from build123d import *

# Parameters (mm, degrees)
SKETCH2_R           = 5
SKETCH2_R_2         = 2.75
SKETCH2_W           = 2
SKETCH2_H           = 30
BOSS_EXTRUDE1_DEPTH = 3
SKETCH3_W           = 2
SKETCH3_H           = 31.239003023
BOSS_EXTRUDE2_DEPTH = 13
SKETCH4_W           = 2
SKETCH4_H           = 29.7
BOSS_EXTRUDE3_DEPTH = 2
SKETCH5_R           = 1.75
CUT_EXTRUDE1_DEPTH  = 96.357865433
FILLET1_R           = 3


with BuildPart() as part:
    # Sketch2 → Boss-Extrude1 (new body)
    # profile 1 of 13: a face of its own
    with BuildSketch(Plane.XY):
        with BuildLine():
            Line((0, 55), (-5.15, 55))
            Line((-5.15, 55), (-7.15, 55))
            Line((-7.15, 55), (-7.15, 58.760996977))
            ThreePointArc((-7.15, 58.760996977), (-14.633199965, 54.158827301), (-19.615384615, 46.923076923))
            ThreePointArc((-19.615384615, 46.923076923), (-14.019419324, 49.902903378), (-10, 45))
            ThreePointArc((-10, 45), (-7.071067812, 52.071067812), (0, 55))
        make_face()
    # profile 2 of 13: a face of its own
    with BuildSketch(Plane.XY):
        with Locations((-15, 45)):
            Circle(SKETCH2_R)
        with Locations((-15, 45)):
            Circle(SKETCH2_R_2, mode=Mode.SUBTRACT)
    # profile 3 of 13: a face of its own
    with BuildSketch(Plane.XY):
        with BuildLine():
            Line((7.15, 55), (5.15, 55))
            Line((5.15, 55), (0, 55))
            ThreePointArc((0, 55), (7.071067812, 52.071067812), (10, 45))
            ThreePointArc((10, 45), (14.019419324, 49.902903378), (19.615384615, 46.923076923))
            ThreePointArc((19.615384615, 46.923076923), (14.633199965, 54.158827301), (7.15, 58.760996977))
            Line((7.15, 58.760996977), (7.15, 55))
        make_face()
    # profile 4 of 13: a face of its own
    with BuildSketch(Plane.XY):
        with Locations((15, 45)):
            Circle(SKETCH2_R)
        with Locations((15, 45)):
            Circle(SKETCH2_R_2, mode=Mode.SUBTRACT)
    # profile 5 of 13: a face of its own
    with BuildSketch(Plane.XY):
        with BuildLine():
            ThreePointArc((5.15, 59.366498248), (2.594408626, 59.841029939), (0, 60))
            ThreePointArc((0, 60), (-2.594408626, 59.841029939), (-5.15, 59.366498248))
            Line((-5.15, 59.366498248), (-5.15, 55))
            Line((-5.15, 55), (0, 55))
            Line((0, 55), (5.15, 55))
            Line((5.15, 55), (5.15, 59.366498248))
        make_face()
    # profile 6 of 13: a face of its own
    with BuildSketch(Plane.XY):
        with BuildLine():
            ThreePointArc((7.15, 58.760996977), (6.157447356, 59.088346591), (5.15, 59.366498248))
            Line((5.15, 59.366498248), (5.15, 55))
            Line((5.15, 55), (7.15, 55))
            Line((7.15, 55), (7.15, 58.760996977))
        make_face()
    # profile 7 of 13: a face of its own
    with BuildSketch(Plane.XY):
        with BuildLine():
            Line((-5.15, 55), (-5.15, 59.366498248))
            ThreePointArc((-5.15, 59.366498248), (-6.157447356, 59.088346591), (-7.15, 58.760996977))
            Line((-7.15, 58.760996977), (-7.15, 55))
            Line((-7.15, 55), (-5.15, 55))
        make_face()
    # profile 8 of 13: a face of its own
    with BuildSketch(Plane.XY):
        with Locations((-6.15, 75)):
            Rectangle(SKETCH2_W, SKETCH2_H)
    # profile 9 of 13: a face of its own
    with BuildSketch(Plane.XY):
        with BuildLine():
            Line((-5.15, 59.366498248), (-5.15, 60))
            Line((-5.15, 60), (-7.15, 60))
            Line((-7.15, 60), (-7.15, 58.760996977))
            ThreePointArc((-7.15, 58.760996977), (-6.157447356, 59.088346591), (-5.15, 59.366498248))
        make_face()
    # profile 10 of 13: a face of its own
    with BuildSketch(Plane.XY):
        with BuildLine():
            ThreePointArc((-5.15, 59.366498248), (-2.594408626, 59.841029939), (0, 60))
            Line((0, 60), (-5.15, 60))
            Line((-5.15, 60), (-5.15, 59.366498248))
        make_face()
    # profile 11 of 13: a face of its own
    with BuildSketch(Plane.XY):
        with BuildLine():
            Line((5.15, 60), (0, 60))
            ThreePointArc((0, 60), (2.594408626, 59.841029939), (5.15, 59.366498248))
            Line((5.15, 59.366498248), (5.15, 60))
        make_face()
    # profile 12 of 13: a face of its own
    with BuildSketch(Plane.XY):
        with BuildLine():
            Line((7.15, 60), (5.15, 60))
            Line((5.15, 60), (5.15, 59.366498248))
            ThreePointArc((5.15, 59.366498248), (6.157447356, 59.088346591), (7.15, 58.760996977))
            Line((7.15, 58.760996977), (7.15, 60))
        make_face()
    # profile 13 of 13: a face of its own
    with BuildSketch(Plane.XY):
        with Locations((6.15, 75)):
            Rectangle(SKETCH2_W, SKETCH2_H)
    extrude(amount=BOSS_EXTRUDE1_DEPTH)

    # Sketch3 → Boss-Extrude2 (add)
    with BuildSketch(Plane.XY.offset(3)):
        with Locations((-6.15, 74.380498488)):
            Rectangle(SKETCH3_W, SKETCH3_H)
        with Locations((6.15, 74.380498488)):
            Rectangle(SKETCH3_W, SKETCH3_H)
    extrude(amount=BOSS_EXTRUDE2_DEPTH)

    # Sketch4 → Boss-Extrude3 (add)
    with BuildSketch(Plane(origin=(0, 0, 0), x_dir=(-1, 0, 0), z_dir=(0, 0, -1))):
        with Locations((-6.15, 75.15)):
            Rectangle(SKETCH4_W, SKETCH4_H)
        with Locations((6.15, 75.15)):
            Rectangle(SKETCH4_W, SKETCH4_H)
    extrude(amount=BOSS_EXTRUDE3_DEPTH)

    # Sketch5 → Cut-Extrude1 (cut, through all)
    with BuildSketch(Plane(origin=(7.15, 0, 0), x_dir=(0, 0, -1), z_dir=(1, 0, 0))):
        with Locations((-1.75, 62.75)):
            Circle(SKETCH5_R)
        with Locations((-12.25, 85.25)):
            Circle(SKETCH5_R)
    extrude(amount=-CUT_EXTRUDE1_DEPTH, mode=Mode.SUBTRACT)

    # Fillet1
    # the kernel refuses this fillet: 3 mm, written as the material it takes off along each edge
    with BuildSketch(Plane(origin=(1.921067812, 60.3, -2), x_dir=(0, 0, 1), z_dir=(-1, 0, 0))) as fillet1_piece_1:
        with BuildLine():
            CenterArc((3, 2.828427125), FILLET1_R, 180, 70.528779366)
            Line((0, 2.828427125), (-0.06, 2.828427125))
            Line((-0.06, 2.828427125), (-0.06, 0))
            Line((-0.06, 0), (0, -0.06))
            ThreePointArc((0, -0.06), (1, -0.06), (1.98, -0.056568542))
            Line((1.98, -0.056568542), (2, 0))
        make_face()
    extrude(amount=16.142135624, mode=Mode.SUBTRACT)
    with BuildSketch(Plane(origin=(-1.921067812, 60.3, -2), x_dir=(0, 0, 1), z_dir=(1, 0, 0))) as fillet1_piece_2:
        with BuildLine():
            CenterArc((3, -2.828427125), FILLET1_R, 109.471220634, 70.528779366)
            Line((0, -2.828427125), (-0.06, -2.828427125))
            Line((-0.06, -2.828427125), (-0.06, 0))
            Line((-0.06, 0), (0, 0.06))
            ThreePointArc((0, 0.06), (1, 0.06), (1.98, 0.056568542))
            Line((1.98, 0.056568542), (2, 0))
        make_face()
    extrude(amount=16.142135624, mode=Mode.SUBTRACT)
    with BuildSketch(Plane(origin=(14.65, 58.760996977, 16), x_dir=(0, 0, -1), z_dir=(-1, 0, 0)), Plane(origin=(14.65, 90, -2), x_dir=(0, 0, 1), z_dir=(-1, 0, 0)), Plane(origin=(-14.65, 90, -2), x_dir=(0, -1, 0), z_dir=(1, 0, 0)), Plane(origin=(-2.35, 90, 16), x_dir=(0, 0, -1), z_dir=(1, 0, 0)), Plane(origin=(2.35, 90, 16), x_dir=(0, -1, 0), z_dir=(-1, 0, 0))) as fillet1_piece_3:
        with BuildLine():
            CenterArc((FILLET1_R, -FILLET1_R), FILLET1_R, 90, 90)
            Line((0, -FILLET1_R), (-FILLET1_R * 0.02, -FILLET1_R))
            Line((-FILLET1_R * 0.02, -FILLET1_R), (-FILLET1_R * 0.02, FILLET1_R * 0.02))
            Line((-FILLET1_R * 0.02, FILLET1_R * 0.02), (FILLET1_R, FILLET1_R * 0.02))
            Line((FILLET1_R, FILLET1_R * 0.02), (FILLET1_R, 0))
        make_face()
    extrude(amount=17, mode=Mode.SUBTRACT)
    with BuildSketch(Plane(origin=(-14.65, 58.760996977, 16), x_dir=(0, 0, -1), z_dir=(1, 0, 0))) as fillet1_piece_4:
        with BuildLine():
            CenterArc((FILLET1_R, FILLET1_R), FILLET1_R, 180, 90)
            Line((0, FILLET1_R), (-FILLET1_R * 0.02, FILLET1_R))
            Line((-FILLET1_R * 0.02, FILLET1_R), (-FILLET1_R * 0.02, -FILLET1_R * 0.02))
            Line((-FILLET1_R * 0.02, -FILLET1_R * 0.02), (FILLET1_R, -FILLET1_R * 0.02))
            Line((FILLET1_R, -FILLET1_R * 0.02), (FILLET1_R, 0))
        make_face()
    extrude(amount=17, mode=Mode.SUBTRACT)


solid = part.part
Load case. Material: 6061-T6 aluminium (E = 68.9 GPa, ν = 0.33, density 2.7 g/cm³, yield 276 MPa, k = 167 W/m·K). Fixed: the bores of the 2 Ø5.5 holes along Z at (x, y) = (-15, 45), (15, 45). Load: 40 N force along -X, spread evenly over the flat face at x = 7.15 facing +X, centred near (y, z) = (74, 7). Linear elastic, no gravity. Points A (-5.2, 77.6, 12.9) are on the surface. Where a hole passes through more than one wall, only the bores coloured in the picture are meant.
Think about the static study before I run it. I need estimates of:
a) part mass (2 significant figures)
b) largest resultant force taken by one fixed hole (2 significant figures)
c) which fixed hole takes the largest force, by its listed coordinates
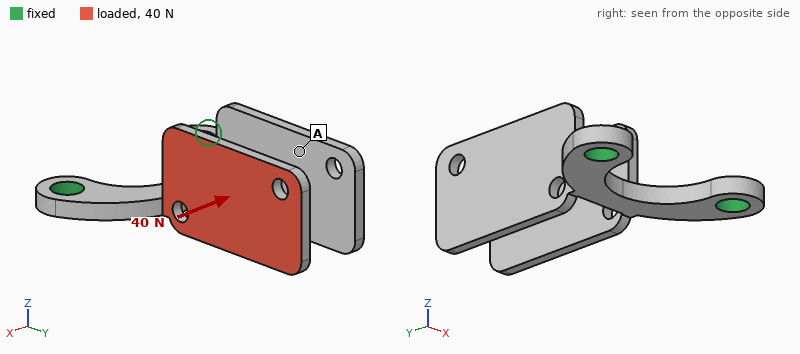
8.4 g
61 N
(-15, 45)
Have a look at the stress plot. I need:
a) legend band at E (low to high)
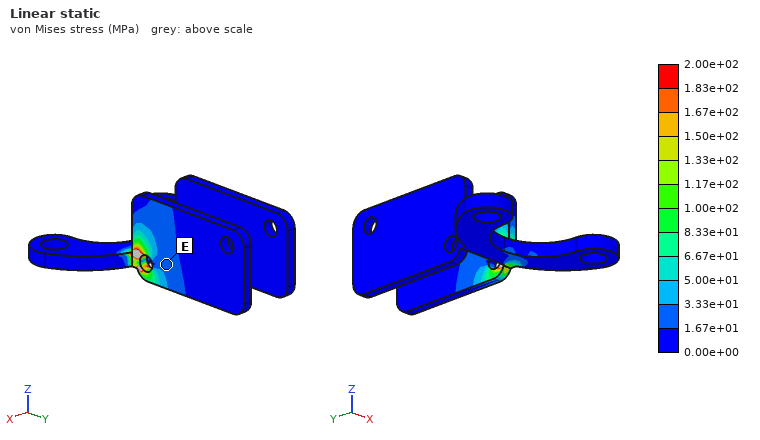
1.67e+01 to 3.33e+01 MPa
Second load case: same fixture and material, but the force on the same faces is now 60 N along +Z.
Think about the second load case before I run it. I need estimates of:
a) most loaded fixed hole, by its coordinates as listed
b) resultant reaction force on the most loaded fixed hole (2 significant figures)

(15, 45)
43 N
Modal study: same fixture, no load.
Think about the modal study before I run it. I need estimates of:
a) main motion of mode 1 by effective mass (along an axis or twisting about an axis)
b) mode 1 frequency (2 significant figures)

along Z
890 Hz
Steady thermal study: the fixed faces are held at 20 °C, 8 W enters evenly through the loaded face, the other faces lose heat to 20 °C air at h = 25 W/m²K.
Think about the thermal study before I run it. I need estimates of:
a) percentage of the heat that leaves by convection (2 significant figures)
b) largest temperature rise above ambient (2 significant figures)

17 %
59 K
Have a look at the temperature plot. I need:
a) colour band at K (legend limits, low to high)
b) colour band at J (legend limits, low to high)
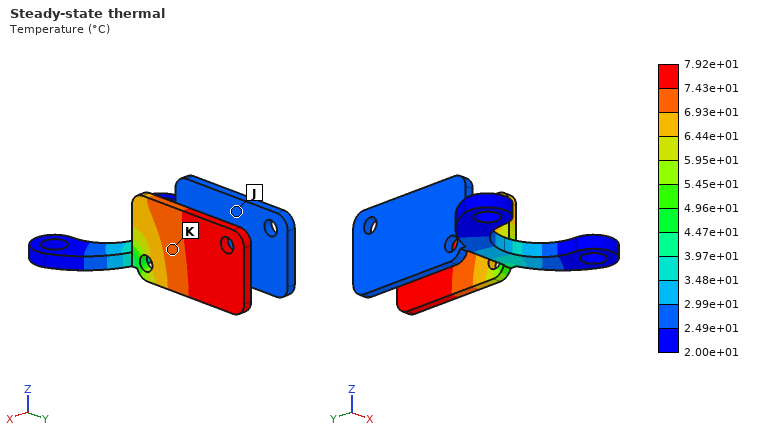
6.93e+01 to 7.43e+01 °C
2.49e+01 to 2.99e+01 °C
